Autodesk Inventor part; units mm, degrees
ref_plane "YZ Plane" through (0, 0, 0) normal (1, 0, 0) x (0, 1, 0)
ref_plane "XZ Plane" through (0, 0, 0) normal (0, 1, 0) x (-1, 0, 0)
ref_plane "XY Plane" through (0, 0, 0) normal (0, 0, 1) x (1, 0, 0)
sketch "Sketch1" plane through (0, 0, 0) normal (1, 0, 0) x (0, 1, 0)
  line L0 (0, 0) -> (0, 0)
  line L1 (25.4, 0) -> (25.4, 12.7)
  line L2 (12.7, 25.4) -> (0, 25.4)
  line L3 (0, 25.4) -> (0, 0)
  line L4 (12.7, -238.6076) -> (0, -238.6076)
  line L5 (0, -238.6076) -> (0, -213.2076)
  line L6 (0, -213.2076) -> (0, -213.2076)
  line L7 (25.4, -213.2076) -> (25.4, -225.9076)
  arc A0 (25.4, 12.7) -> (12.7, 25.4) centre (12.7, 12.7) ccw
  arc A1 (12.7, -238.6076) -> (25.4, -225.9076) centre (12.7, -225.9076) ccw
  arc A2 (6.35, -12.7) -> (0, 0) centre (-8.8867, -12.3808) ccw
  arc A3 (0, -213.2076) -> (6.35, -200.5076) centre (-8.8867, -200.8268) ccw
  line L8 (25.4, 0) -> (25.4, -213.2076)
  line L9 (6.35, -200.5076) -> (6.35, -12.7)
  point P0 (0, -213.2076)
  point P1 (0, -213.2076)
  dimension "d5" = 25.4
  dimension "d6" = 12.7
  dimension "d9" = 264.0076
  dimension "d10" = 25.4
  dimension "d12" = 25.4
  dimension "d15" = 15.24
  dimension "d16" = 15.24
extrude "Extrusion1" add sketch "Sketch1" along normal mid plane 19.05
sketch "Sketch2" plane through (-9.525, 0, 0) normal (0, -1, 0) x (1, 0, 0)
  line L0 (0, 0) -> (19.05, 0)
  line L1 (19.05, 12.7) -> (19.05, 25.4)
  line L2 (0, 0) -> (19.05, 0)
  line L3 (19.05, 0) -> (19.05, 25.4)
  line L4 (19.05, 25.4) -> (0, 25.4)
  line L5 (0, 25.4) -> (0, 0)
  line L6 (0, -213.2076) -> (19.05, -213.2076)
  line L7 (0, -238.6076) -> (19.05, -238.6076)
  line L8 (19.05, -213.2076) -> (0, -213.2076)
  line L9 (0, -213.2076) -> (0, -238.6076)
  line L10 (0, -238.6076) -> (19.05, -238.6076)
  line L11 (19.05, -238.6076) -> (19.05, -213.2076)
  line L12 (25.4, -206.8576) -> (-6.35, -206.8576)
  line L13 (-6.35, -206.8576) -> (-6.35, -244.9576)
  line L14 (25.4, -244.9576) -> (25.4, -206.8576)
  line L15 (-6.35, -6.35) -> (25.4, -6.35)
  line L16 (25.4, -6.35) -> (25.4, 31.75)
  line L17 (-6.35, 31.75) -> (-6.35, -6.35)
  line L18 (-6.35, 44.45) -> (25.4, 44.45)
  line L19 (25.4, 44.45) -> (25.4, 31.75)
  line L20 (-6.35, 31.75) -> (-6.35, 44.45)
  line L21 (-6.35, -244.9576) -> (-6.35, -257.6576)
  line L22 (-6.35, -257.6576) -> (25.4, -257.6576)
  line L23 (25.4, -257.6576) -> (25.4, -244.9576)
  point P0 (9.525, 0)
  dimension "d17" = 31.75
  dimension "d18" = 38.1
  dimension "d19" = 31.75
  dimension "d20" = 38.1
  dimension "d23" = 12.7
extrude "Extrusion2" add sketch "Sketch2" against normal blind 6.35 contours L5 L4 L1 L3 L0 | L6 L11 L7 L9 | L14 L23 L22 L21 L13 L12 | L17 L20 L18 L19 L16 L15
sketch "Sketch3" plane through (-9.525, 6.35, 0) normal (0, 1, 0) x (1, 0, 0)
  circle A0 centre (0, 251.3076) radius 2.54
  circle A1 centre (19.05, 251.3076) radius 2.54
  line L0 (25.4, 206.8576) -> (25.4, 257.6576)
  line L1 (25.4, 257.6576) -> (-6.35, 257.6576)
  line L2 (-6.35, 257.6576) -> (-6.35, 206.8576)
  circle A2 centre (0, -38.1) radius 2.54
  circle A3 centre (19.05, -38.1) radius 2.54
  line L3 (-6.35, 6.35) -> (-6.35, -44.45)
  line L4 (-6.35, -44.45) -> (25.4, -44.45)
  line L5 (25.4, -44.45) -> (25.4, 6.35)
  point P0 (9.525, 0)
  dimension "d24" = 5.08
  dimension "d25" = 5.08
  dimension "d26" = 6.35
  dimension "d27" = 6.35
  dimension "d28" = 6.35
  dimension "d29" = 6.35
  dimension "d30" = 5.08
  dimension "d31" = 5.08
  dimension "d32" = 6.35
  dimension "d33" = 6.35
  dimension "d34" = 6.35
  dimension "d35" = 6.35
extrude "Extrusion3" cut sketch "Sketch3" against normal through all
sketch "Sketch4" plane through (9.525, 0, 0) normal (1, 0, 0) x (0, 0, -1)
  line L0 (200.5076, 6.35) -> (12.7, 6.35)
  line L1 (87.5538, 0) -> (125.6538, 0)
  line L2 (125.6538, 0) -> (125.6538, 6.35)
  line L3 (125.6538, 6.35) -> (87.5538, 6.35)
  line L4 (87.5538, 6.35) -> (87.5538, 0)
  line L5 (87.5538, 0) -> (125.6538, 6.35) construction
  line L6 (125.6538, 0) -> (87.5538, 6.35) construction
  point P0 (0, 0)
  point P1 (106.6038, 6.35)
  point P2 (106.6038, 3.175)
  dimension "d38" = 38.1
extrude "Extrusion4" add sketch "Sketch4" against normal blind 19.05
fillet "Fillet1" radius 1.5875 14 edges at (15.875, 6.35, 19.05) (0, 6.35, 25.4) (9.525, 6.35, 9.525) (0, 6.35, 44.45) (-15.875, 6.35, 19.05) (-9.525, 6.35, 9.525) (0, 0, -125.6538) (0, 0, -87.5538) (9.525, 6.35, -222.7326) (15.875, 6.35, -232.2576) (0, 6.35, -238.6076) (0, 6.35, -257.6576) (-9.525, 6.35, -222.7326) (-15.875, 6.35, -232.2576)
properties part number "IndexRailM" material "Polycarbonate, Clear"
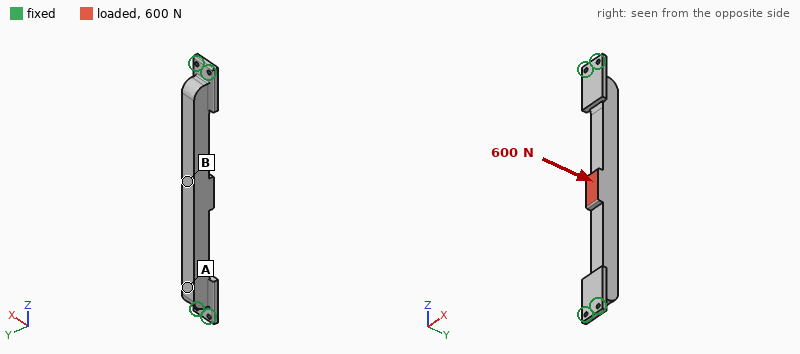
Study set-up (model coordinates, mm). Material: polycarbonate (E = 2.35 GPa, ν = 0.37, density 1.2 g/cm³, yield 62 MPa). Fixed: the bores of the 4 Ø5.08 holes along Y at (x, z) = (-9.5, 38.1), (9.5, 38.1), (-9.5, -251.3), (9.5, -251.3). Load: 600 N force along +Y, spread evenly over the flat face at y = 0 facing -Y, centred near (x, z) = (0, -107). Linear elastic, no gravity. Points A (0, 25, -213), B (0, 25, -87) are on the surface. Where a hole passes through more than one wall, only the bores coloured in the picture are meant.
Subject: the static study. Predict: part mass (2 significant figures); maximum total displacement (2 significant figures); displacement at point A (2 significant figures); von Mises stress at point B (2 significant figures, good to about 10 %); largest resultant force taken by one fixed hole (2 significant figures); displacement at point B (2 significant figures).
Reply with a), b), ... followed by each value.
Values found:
a) 140 g
b) 2.8 mm
c) 0.77 mm
d) 17 MPa
e) 690 N
f) 2.7 mm
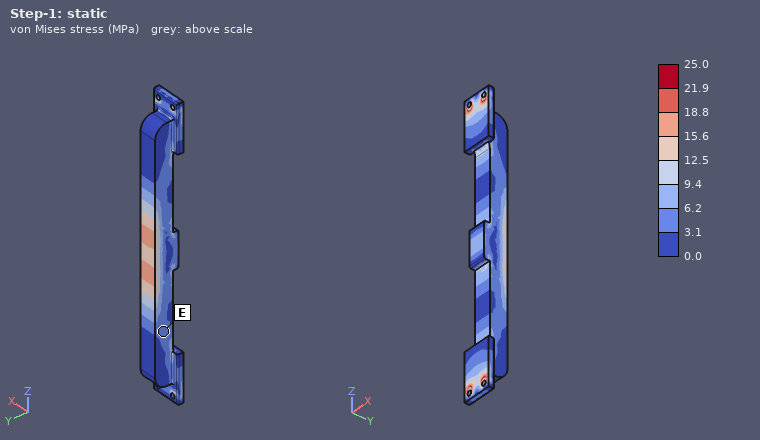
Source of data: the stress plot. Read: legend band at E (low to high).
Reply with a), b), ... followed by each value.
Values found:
a) 3.1 to 6.2 MPa
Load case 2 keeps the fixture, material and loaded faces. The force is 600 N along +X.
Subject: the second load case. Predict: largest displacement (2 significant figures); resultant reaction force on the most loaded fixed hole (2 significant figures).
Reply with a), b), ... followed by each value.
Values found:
a) 3.0 mm
b) 1.1 kN
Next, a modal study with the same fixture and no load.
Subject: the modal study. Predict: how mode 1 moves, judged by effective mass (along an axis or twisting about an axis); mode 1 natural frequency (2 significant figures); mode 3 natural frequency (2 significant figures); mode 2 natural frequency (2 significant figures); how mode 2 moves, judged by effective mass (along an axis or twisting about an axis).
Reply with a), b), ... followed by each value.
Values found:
a) along Y
b) 300 Hz
c) 600 Hz
d) 330 Hz
e) along X
